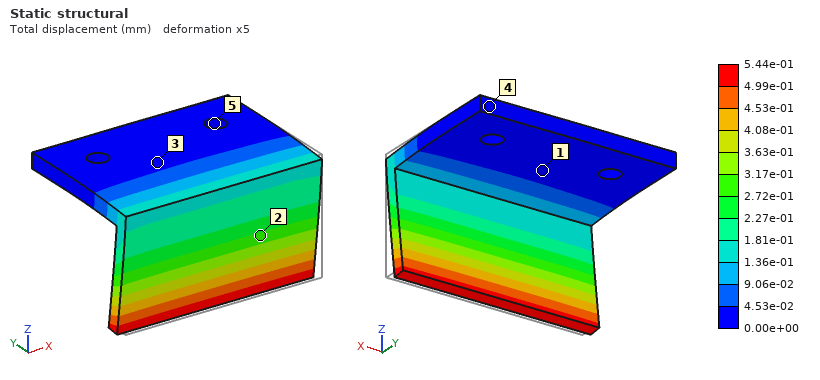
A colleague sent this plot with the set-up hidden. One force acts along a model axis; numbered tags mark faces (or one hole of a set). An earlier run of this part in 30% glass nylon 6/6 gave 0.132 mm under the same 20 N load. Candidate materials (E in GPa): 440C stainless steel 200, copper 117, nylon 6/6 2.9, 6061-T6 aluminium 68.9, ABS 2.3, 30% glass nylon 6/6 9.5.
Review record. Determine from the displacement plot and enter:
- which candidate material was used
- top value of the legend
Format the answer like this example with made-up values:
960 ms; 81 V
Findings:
ABS; 5.44e-01 mm
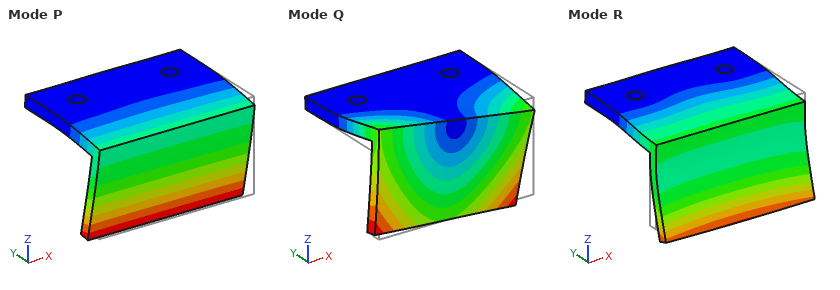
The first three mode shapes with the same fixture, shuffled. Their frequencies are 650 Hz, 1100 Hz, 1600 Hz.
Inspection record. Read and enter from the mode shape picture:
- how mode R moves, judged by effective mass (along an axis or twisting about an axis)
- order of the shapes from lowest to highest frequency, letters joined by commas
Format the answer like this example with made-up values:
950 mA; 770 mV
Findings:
along Z; P, Q, R
